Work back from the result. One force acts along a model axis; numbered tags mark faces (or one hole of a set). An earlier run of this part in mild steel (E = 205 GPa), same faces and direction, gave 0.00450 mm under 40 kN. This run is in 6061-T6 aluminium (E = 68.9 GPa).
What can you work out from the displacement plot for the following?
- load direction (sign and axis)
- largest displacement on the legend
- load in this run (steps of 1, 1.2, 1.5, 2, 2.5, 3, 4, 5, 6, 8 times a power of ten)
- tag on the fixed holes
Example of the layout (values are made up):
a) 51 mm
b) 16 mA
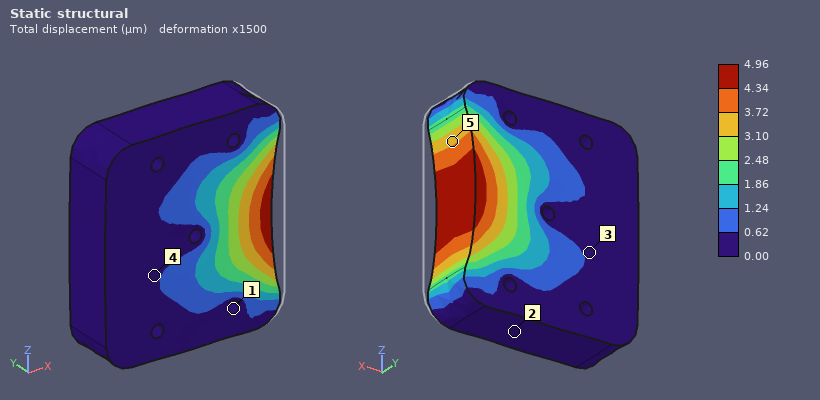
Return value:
a) -X
b) 4.96 µm
c) 15 kN
d) 1
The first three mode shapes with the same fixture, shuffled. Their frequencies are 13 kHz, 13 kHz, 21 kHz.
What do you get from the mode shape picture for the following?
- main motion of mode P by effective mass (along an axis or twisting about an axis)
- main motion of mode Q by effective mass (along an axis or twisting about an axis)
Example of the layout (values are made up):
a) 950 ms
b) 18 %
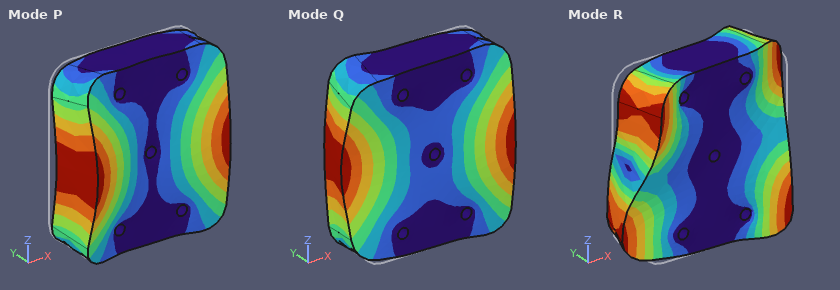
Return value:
a) along Y
b) twisting about Z
